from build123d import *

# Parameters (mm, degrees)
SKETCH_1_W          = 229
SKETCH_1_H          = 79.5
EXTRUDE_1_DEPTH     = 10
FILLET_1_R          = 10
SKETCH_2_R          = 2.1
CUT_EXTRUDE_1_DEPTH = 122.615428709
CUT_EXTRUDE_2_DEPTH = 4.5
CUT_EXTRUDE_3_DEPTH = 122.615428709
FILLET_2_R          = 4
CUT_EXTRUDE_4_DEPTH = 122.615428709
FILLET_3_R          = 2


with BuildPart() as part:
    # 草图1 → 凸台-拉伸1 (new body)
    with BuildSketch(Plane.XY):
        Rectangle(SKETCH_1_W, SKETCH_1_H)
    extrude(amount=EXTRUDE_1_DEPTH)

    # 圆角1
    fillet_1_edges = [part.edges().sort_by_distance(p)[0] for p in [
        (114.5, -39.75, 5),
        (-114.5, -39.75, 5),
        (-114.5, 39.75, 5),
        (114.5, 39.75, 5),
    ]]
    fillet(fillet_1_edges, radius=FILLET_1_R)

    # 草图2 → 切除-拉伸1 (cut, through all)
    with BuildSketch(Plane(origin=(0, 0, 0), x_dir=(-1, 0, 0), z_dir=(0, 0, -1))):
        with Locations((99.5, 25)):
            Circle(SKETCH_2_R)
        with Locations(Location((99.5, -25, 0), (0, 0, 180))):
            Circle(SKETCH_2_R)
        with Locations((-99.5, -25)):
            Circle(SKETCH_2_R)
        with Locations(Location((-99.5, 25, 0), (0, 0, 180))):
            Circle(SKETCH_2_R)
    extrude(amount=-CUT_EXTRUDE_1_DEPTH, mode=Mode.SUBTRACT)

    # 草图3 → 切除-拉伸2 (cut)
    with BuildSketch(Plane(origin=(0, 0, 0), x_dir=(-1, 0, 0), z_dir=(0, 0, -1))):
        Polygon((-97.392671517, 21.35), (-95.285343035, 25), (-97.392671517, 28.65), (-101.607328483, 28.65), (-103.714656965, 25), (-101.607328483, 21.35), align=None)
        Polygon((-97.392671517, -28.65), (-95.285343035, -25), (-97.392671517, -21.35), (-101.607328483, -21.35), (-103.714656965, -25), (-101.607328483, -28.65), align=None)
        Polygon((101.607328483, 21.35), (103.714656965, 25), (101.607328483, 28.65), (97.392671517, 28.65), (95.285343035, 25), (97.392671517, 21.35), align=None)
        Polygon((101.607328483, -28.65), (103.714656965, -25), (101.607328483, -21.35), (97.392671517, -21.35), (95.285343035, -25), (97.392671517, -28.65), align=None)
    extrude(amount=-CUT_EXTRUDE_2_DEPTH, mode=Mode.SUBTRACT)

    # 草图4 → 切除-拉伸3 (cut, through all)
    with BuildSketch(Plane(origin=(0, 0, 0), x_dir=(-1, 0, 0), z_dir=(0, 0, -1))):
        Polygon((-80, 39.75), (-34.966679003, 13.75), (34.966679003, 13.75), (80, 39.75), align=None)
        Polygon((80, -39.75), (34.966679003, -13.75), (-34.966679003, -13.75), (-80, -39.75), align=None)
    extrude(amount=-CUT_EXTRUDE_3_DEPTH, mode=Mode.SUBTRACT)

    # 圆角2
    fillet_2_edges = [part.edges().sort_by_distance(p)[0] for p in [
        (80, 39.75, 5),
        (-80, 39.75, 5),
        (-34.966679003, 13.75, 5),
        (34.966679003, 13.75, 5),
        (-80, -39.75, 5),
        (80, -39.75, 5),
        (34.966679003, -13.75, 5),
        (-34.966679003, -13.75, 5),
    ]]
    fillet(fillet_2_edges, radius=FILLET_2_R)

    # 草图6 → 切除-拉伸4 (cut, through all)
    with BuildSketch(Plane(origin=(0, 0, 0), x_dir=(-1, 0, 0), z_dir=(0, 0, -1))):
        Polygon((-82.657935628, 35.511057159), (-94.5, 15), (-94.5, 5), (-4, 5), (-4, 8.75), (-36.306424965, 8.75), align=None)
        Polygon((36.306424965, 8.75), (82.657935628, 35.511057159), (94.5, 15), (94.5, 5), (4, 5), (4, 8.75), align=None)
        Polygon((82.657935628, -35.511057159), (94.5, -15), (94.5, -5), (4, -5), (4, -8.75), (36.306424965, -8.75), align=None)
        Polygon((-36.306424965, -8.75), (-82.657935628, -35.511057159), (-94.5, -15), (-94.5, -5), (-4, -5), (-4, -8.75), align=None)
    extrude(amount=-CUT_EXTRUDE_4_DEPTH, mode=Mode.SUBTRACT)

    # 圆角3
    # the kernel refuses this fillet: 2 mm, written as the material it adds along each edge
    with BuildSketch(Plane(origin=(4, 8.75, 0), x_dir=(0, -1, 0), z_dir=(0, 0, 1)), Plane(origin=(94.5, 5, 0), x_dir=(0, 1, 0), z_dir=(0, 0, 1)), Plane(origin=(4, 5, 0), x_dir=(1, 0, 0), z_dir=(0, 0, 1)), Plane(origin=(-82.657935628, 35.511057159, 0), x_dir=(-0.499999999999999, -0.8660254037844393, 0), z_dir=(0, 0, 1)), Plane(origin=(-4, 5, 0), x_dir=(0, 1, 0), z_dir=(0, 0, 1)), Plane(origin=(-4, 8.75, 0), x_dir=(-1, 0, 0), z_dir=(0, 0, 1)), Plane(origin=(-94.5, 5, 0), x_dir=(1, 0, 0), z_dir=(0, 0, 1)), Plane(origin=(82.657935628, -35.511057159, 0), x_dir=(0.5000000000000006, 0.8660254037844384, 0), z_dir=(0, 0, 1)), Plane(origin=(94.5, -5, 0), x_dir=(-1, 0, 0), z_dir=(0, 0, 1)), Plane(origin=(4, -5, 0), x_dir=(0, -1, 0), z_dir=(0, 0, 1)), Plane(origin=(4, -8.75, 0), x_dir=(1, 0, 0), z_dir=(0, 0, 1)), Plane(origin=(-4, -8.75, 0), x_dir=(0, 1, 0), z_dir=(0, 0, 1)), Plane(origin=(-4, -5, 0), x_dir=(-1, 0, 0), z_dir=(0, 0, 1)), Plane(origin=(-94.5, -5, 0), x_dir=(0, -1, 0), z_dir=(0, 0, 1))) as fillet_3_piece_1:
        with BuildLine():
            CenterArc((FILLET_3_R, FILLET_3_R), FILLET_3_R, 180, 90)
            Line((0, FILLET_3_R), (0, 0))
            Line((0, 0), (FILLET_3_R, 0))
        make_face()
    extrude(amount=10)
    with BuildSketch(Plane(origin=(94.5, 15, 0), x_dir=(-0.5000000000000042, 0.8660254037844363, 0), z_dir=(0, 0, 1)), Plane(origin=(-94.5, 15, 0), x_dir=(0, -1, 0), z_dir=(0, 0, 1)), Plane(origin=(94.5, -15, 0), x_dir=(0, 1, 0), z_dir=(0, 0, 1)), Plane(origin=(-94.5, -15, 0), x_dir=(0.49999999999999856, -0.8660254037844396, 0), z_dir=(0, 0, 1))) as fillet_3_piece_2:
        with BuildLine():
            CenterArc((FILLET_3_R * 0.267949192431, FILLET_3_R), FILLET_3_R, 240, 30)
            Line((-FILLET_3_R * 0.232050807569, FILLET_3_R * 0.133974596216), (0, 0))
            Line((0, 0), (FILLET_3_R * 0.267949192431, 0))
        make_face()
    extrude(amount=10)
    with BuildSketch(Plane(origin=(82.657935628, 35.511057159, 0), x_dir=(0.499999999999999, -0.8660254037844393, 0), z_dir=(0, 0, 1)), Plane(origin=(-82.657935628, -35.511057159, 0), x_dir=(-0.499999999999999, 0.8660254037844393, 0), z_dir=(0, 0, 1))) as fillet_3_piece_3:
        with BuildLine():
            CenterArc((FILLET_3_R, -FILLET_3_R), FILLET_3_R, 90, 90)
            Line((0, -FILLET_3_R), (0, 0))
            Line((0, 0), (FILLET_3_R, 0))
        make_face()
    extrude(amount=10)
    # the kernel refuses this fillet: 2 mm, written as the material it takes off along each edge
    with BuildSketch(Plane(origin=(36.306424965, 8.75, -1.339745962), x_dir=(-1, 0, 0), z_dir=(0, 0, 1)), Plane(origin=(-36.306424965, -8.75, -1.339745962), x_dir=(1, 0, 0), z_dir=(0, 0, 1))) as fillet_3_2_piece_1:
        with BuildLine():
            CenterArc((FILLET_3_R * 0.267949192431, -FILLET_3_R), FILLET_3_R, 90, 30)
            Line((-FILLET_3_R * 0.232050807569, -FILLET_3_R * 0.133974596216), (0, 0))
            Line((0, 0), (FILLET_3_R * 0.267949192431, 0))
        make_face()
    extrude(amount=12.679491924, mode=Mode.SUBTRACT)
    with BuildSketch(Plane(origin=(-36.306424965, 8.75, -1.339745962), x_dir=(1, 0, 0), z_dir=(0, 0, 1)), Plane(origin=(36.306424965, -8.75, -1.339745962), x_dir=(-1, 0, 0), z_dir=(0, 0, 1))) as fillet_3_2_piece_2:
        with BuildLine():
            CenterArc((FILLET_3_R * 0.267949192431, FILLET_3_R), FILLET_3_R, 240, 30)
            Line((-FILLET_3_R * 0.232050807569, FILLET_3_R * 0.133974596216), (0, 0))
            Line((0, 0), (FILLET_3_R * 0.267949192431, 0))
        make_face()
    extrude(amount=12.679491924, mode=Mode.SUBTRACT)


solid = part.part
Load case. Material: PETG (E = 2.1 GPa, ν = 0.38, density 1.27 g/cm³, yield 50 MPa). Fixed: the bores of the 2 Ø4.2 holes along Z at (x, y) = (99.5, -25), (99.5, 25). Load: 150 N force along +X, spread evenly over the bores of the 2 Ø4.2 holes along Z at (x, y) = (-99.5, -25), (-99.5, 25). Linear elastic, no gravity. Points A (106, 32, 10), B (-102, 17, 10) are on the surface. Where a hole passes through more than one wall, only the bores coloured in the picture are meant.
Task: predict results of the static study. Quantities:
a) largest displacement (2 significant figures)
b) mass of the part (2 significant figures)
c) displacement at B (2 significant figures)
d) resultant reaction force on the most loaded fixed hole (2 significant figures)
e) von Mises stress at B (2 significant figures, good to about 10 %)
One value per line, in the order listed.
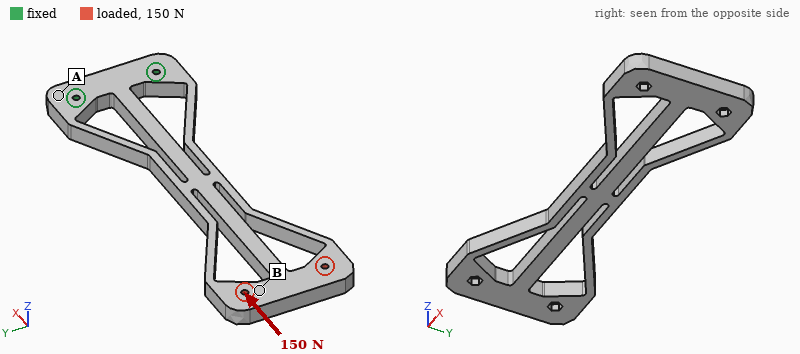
2.4 mm
94 g
2.1 mm
77 N
0.89 MPa
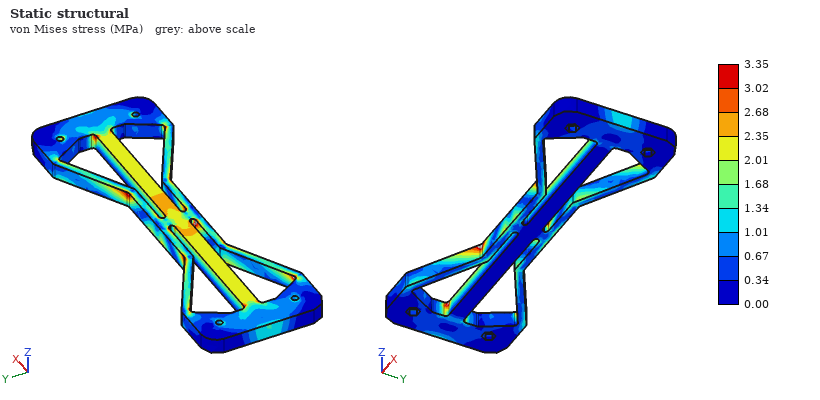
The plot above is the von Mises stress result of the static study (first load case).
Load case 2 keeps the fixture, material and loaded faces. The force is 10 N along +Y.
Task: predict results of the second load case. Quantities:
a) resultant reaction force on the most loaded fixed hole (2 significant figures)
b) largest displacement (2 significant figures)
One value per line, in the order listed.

37 N
2.9 mm
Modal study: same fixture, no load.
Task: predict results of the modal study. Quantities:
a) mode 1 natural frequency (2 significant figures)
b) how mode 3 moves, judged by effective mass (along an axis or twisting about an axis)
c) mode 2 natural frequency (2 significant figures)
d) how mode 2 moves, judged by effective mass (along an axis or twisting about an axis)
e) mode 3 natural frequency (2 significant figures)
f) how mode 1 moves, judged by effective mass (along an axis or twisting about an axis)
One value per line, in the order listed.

29 Hz
twisting about X
56 Hz
along Y
120 Hz
along Z
